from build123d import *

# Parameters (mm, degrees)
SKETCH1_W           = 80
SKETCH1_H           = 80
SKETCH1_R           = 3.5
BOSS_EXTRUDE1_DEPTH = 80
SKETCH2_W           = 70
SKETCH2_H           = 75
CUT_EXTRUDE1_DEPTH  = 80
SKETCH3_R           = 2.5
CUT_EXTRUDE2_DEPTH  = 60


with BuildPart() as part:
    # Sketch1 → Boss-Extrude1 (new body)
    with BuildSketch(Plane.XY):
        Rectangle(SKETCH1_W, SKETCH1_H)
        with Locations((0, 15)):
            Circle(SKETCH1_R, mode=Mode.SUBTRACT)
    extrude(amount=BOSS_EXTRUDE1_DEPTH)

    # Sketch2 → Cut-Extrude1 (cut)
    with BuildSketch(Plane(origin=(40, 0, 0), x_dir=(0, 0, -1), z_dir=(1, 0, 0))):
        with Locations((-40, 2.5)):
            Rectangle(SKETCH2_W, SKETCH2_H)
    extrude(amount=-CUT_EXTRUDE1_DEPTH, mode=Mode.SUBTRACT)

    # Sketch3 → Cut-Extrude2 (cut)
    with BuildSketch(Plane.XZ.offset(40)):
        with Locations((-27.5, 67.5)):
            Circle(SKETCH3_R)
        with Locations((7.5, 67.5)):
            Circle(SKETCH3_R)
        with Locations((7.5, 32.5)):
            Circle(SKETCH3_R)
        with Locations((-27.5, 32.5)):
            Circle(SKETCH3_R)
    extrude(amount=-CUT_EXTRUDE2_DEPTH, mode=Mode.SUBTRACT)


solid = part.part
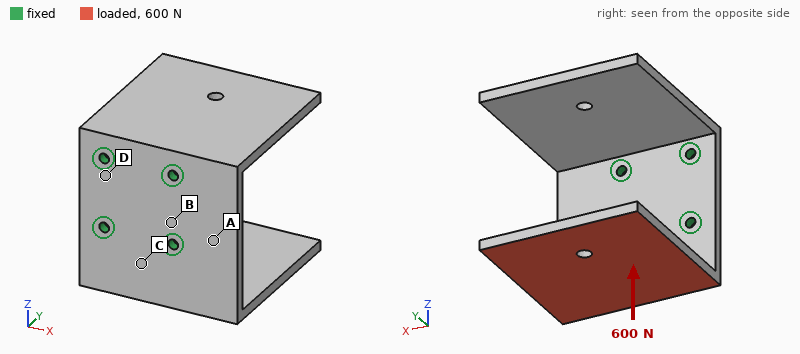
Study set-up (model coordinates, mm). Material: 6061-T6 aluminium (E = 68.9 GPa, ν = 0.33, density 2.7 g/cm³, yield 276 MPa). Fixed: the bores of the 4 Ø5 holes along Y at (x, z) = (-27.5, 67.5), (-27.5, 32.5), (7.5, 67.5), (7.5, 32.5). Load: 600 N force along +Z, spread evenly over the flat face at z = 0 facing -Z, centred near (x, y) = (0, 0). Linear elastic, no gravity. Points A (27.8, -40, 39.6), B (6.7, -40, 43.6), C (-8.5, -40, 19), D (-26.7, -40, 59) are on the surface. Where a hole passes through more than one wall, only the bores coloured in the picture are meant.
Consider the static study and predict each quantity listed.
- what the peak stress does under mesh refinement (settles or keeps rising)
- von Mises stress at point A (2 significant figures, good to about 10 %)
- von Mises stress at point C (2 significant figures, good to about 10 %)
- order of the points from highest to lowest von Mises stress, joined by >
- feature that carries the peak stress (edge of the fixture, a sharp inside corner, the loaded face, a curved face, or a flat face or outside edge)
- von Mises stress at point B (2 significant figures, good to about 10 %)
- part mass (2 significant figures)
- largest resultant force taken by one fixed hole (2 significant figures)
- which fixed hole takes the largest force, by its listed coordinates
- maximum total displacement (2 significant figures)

keeps rising
24 MPa
60 MPa
C > A > B > D
edge of the fixture
11 MPa
250 g
400 N
(7.5, 32.5)
1.4 mm
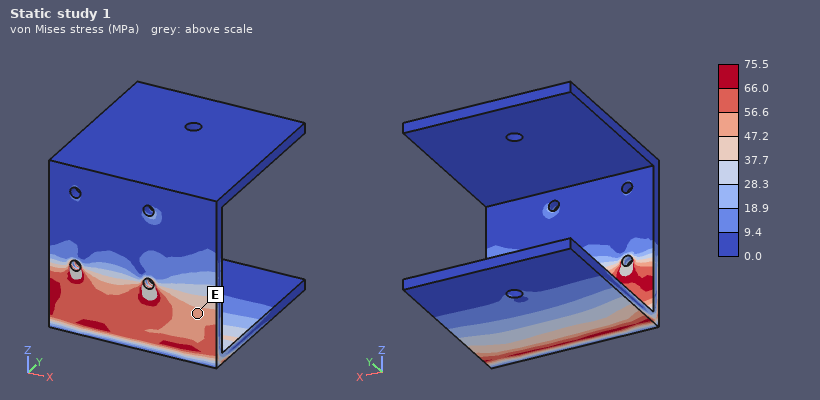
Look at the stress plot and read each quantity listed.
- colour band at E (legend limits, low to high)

47.2 to 56.6 MPa
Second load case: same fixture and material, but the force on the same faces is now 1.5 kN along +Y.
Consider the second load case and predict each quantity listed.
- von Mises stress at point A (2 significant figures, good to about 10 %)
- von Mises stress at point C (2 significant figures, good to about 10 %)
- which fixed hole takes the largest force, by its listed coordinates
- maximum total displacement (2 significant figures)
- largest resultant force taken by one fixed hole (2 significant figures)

51 MPa
81 MPa
(7.5, 32.5)
1.3 mm
1.4 kN
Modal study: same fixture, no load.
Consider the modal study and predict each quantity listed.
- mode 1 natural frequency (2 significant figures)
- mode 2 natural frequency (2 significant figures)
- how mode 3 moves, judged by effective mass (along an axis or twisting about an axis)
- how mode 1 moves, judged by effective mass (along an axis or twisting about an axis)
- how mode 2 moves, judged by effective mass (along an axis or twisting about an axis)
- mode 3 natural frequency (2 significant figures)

430 Hz
570 Hz
along X
along Z
along Z
850 Hz
